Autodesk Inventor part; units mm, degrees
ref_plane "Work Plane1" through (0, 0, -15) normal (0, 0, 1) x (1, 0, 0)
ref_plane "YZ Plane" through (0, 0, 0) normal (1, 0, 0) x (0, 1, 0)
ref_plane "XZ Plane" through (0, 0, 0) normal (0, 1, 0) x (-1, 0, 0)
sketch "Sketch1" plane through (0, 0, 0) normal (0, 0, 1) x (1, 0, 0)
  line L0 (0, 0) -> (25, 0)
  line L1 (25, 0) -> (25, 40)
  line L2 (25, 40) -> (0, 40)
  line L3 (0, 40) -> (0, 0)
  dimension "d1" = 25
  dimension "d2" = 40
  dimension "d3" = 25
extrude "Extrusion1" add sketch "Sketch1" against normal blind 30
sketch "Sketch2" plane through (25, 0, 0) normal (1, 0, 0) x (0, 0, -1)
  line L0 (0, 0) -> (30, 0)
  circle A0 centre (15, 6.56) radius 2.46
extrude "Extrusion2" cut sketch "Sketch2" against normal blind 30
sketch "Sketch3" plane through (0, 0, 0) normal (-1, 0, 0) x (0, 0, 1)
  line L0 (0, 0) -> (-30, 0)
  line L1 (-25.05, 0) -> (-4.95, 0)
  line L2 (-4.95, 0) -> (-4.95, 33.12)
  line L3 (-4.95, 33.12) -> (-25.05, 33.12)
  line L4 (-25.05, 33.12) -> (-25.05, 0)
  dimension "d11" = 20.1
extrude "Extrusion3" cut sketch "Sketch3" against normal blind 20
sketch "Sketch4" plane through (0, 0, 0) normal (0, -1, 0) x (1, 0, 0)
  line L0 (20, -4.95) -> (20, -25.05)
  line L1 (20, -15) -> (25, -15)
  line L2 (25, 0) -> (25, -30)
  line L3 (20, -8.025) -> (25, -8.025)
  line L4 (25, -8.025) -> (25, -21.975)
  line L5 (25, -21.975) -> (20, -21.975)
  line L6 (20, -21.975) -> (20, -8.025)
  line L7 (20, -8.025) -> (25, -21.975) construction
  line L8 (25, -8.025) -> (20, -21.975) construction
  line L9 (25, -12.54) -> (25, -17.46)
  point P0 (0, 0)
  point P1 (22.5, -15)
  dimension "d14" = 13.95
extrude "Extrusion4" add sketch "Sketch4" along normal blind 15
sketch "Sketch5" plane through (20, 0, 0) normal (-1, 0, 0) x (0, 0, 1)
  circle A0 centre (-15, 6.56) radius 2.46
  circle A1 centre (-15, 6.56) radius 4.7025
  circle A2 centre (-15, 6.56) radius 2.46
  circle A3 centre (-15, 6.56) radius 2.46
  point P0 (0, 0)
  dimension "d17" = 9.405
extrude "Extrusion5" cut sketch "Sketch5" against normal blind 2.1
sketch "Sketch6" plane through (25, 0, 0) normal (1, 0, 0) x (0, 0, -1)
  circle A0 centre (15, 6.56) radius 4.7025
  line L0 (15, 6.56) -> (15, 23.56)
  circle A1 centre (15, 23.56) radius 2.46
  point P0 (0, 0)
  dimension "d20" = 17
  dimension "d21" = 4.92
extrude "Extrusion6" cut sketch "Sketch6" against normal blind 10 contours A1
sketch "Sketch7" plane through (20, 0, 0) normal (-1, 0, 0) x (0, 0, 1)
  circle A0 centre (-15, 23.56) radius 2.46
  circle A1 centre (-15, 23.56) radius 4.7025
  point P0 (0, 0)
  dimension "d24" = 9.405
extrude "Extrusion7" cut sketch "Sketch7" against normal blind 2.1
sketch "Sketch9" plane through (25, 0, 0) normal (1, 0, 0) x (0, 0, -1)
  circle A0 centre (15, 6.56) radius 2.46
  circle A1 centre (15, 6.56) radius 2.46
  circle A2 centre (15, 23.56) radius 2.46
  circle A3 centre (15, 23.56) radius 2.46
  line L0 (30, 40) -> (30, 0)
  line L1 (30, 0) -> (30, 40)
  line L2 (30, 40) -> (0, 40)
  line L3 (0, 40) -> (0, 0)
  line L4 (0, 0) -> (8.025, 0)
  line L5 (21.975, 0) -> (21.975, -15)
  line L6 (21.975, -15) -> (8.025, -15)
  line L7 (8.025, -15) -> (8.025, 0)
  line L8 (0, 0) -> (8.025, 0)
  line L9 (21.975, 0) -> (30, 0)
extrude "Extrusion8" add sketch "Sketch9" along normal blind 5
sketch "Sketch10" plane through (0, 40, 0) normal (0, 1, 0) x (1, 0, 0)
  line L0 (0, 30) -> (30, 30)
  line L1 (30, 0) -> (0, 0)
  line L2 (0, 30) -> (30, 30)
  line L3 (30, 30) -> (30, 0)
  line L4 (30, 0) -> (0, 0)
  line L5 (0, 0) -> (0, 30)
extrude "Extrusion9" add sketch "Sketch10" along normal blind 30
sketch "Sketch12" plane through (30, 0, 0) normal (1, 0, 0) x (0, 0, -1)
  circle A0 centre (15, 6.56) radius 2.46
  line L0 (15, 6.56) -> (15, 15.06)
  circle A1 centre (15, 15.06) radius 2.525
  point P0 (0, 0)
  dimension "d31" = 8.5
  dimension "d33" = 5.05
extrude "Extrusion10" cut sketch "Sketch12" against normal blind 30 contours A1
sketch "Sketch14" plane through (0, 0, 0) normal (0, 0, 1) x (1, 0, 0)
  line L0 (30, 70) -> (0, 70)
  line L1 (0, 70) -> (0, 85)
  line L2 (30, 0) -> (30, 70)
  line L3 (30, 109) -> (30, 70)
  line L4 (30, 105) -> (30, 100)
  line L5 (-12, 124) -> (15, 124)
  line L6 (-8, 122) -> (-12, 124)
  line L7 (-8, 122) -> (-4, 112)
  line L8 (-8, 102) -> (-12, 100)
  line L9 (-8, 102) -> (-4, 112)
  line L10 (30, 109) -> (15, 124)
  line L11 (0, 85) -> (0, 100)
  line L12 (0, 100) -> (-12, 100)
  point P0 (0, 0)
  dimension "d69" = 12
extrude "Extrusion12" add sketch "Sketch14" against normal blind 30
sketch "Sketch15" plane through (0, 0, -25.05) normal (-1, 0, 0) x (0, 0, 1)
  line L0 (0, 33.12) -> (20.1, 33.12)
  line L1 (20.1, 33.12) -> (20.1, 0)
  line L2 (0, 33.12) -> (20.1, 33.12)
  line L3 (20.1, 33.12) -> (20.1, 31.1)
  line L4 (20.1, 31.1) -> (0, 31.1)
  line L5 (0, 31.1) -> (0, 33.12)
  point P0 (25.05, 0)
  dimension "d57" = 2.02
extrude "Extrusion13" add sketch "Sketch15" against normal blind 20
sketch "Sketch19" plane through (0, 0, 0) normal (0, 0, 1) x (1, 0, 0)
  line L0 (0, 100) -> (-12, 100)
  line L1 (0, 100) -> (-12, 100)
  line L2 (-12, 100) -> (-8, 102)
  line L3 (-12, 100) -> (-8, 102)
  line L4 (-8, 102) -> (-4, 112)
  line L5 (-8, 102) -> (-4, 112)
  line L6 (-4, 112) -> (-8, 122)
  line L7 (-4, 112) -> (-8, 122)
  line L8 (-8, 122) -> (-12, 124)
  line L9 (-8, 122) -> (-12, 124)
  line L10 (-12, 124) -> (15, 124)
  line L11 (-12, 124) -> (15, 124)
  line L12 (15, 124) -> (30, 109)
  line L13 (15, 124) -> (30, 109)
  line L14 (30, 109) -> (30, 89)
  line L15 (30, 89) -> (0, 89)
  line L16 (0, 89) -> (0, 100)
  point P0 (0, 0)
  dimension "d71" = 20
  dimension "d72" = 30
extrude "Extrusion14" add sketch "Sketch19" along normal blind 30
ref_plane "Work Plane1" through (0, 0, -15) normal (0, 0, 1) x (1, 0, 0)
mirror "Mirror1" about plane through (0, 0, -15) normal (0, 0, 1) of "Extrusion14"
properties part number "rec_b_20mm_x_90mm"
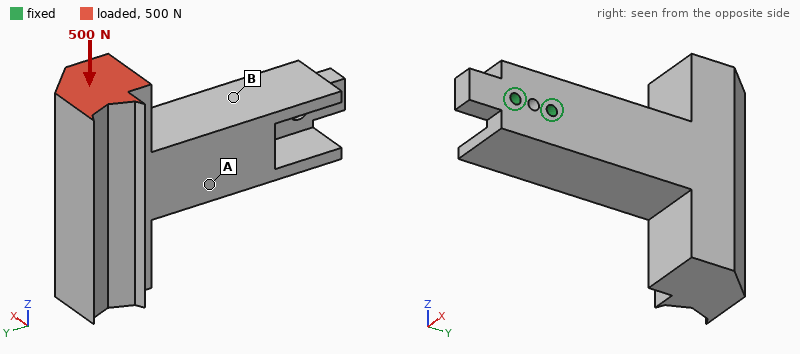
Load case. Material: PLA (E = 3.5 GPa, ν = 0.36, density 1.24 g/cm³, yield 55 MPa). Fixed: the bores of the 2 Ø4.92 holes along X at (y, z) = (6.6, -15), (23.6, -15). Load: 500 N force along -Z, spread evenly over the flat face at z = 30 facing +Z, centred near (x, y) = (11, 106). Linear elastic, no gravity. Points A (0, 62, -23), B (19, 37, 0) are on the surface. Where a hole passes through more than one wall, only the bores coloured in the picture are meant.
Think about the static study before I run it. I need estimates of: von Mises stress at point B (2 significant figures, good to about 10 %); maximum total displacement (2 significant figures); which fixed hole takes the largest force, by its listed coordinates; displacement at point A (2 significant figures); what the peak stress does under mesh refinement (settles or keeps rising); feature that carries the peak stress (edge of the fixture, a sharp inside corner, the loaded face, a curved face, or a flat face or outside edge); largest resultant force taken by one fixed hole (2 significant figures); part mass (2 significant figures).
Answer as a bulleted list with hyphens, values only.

- 11 MPa
- 2.0 mm
- (23.6, -15)
- 0.62 mm
- keeps rising
- edge of the fixture
- 2.3 kN
- 210 g
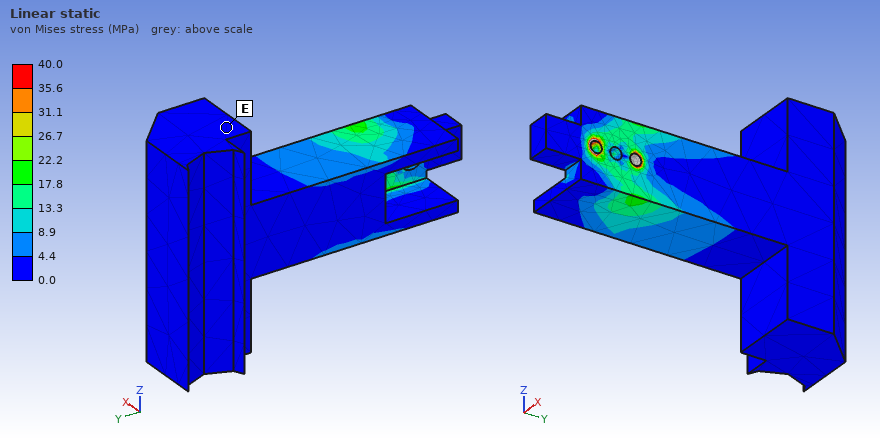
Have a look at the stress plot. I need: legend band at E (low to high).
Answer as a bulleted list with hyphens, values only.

- 0.0 to 4.4 MPa
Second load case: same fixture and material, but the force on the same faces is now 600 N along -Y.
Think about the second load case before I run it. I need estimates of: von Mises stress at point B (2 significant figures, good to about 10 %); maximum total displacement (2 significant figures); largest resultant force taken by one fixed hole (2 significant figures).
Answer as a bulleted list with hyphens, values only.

- 10 MPa
- 1.7 mm
- 1.3 kN
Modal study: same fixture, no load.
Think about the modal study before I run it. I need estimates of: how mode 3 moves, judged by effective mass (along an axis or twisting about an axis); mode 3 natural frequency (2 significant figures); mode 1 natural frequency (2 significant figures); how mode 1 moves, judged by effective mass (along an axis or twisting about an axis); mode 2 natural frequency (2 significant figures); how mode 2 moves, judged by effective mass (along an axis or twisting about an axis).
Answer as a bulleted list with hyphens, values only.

- twisting about Y
- 430 Hz
- 220 Hz
- along X
- 240 Hz
- along Z
